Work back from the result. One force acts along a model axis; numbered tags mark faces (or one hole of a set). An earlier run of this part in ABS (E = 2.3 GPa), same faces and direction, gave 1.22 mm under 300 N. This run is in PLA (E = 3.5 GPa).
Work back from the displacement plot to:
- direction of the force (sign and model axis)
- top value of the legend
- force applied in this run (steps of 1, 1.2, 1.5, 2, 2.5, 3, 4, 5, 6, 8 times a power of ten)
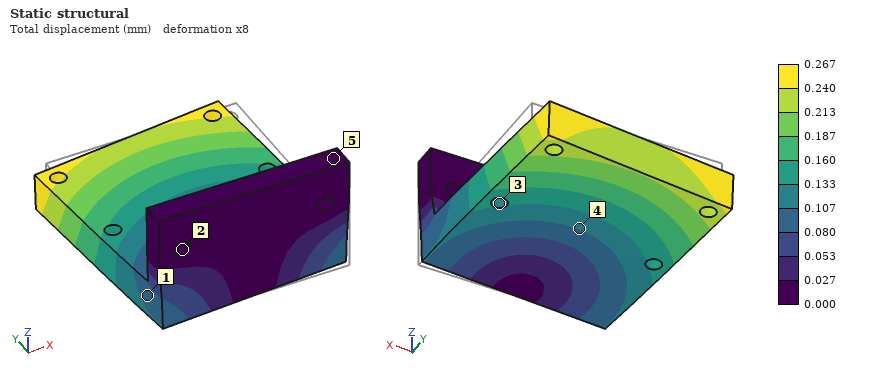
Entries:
-X
0.267 mm
100 N
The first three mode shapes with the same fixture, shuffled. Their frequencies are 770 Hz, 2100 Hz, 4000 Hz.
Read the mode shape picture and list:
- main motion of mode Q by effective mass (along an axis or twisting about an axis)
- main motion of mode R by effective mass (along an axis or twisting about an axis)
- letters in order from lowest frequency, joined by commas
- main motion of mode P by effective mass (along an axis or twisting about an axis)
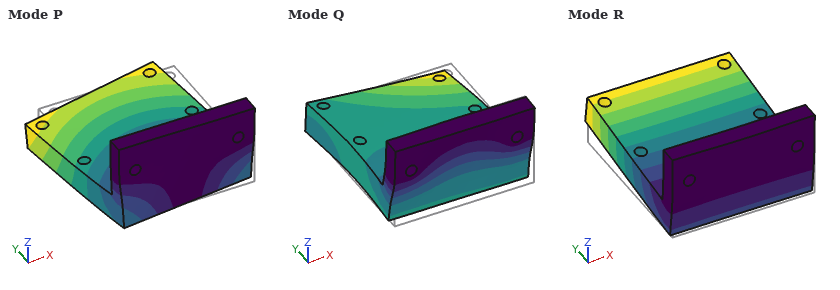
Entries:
along Y
along Z
R, P, Q
along X
